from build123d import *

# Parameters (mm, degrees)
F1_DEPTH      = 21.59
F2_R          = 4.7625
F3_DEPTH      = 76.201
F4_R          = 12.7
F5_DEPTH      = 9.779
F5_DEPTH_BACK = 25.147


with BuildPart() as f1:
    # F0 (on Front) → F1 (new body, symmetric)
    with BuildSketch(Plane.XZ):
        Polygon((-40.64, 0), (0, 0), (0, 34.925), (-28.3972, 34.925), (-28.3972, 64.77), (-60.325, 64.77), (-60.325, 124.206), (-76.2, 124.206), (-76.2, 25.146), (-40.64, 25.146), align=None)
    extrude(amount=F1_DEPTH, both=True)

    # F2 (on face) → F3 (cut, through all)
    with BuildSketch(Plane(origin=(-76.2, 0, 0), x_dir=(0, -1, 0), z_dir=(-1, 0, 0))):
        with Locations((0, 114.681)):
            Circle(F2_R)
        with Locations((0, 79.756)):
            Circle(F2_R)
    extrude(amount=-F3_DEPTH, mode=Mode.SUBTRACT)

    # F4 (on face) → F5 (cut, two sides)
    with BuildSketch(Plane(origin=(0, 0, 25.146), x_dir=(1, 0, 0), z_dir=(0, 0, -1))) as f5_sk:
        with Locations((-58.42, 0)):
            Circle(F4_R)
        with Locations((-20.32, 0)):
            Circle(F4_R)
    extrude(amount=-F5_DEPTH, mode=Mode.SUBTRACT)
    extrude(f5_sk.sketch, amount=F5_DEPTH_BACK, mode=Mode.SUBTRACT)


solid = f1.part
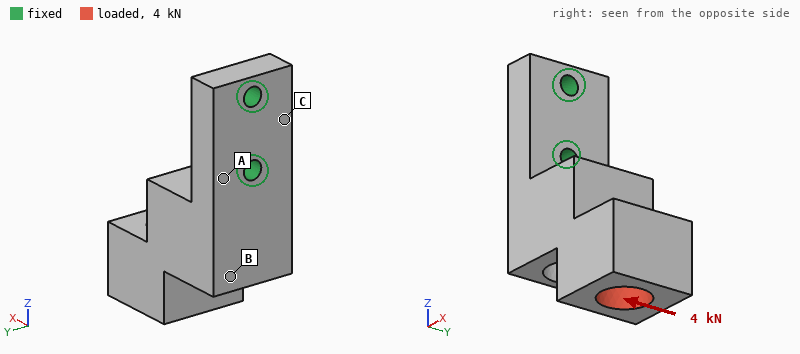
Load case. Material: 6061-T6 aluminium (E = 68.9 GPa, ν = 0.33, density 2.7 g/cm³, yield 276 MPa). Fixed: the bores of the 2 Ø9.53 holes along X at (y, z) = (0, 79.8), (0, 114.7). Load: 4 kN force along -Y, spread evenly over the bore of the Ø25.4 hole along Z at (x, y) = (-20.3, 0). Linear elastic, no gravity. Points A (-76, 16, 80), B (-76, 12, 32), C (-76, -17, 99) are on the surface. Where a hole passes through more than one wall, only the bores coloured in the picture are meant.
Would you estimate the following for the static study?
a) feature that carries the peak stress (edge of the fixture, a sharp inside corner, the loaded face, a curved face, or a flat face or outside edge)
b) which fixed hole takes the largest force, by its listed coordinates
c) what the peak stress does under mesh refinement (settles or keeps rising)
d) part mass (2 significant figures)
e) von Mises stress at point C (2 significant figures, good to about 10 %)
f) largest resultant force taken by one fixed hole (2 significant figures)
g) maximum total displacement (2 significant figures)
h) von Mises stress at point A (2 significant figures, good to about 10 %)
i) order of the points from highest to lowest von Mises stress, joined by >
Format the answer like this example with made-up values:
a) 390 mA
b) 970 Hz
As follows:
a) edge of the fixture
b) (0, 79.8)
c) keeps rising
d) 420 g
e) 30 MPa
f) 8.9 kN
g) 0.35 mm
h) 59 MPa
i) A > C > B
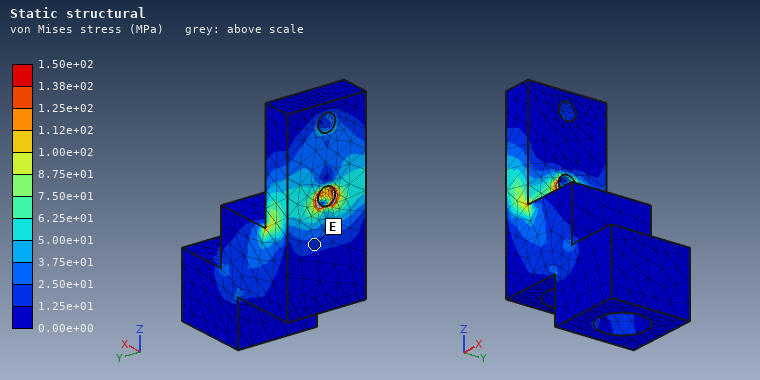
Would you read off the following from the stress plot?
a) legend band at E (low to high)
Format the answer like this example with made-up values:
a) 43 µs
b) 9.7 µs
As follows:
a) 1.25e+01 to 2.50e+01 MPa
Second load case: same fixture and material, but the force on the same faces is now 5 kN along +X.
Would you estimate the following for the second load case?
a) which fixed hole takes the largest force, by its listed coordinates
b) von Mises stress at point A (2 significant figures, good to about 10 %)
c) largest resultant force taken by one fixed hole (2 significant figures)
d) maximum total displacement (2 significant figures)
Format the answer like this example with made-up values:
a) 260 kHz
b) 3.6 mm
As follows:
a) (0, 79.8)
b) 89 MPa
c) 7.7 kN
d) 0.76 mm
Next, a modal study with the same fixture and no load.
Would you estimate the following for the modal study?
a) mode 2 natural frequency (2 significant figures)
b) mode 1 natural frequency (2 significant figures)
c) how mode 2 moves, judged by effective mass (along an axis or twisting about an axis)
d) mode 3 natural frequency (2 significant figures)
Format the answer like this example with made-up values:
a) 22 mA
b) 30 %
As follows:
a) 1600 Hz
b) 1100 Hz
c) along Y
d) 4100 Hz
